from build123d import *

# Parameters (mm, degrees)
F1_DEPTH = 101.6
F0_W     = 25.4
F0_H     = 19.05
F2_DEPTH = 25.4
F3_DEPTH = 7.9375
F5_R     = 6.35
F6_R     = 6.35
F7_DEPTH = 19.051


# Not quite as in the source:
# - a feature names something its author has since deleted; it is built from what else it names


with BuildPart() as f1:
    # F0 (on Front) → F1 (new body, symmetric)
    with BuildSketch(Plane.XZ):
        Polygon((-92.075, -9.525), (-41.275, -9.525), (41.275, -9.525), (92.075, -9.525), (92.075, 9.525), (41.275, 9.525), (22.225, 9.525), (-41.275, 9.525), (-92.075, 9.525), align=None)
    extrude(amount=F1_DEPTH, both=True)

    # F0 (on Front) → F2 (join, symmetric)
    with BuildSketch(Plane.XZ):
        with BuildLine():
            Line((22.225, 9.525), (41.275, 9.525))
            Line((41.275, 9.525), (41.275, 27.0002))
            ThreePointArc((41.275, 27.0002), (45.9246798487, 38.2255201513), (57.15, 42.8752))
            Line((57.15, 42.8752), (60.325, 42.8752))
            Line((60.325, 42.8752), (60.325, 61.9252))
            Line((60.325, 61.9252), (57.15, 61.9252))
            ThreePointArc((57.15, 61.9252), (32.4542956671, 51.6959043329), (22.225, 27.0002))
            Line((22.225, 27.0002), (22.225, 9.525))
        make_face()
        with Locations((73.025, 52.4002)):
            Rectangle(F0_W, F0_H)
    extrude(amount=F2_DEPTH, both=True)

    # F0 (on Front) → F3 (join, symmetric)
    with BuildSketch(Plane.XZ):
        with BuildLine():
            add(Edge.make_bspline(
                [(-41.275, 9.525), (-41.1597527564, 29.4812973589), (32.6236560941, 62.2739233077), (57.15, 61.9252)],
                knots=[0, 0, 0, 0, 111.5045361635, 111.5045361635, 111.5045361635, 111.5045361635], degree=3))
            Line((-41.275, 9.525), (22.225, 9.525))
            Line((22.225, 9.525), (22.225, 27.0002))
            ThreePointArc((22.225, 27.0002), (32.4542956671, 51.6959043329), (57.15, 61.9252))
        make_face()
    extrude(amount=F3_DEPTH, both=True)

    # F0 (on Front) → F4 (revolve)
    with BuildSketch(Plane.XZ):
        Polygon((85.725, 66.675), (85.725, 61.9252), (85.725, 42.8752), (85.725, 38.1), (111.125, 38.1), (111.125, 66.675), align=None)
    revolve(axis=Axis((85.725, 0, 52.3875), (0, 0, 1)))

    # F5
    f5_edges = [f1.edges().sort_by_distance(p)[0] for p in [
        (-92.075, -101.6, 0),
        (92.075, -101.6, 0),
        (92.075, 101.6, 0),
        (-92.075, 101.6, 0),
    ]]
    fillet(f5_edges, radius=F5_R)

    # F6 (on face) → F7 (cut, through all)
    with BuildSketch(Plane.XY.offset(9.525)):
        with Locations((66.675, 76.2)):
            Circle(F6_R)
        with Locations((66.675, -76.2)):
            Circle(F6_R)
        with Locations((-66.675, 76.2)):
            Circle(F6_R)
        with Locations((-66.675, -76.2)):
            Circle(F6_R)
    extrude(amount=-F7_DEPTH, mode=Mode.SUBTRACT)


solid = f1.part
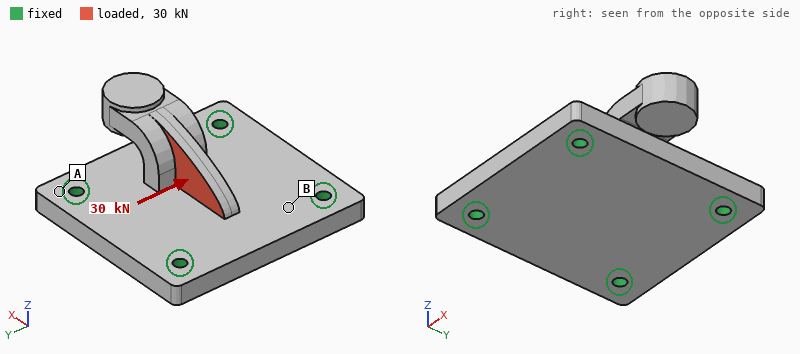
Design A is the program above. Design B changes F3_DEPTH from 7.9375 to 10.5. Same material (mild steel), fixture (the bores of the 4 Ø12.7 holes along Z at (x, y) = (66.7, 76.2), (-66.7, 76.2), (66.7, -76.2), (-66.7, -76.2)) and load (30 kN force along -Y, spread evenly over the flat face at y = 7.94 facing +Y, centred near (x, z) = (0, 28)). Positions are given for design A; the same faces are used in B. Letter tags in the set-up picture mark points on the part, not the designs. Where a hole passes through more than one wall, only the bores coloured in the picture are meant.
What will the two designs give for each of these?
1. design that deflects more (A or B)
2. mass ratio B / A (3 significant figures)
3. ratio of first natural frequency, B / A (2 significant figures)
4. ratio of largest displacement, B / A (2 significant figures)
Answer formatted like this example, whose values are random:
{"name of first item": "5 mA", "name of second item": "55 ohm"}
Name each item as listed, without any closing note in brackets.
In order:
{"design that deflects more": "A", "mass ratio B / A": "1.01", "ratio of first natural frequency, B / A": "1.0", "ratio of largest displacement, B / A": "0.82"}
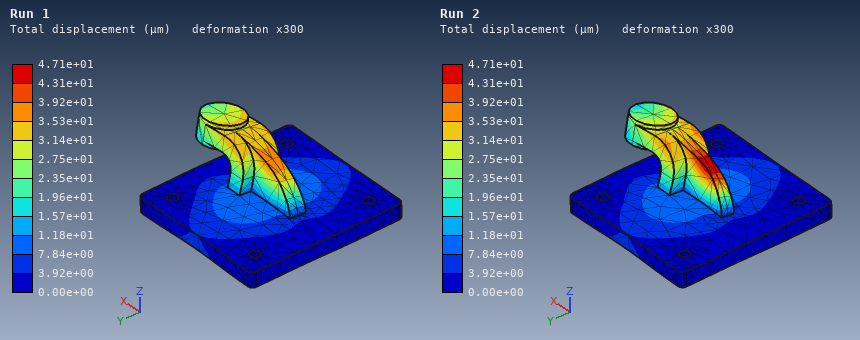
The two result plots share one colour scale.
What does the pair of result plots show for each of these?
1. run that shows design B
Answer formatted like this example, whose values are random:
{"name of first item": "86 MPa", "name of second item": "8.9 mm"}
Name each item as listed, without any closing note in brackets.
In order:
{"run that shows design B": "Run 1"}
